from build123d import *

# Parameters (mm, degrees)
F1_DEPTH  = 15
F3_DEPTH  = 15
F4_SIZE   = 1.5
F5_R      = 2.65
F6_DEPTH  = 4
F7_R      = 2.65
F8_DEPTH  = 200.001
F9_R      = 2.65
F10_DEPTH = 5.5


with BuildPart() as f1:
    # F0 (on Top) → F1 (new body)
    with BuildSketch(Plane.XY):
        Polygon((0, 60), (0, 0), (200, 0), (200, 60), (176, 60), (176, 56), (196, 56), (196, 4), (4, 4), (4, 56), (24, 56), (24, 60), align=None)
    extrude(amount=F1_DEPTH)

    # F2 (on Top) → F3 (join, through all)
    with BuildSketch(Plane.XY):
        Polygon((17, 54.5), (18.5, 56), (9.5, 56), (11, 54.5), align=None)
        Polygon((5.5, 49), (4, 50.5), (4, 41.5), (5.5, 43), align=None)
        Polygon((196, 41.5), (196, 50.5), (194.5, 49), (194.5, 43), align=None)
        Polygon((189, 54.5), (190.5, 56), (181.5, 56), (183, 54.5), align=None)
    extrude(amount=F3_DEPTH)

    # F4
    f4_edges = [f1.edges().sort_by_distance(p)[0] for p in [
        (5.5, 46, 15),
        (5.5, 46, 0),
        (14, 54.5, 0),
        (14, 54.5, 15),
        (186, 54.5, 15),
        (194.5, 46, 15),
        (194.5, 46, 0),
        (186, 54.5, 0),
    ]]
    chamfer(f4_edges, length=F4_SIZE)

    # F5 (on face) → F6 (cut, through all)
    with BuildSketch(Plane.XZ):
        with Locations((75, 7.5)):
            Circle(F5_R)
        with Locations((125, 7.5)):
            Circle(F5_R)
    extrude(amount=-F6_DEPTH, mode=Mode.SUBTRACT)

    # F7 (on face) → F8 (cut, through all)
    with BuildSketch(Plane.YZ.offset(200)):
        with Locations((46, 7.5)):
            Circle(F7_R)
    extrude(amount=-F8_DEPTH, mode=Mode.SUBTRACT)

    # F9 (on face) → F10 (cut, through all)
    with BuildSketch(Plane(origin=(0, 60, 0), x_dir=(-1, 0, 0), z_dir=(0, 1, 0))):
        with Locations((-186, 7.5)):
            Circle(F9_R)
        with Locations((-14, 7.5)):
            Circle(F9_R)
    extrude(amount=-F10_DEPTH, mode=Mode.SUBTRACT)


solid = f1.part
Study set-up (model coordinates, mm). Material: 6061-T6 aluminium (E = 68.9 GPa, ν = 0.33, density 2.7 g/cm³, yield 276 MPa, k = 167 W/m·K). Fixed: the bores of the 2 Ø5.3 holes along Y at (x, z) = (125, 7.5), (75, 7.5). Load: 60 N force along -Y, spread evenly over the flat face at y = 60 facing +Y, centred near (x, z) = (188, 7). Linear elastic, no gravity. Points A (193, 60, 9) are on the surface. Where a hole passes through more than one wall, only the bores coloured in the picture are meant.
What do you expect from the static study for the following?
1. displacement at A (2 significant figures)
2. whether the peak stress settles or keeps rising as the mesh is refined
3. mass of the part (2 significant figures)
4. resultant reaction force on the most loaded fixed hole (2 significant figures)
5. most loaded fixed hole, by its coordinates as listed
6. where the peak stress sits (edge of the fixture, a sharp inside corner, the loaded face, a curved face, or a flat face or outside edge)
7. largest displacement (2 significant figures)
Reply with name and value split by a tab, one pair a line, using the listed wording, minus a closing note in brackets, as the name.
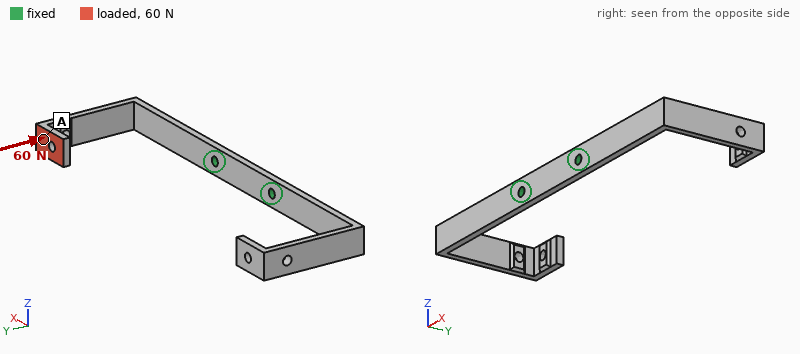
displacement at A	1.4 mm
whether the peak stress settles or keeps rising as the mesh is refined	keeps rising
mass of the part	57 g
resultant reaction force on the most loaded fixed hole	60 N
most loaded fixed hole, by its coordinates as listed	(125, 7.5)
where the peak stress sits	edge of the fixture
largest displacement	1.5 mm
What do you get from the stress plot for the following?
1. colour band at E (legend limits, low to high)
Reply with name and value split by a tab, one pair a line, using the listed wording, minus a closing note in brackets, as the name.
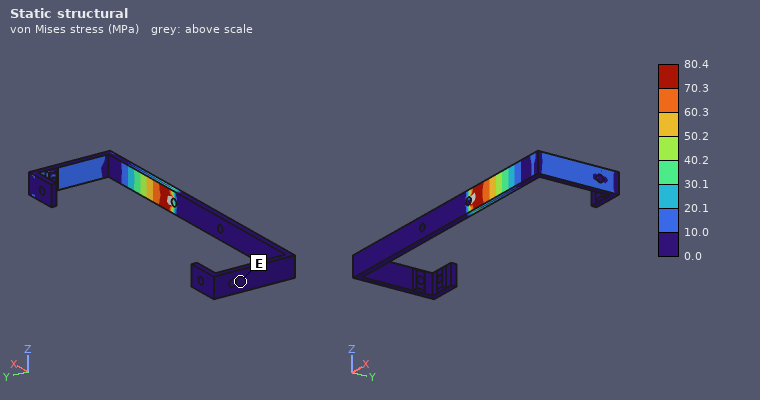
colour band at E	0.0 to 10.0 MPa
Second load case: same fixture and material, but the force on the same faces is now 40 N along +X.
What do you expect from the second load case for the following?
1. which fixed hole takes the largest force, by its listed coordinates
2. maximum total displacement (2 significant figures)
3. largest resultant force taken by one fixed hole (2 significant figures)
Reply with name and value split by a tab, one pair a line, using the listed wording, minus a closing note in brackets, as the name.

which fixed hole takes the largest force, by its listed coordinates	(125, 7.5)
maximum total displacement	2.4 mm
largest resultant force taken by one fixed hole	39 N
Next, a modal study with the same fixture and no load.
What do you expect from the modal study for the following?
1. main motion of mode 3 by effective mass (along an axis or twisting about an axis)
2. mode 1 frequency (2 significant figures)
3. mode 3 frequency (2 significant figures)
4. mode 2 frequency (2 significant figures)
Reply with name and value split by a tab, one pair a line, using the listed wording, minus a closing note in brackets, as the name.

main motion of mode 3 by effective mass	along Z
mode 1 frequency	210 Hz
mode 3 frequency	340 Hz
mode 2 frequency	210 Hz
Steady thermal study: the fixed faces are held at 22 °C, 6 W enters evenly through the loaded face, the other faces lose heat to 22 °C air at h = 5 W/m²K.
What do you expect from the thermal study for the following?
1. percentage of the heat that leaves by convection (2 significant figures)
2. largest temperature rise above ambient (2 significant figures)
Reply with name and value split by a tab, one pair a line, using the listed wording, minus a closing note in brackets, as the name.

percentage of the heat that leaves by convection	17 %
largest temperature rise above ambient	72 K
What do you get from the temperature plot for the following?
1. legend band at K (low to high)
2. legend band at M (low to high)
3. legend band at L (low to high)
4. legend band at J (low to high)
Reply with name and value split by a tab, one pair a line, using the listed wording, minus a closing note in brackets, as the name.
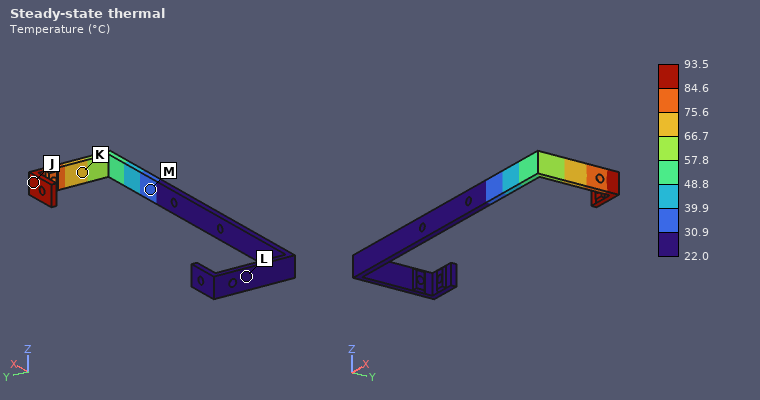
legend band at K	66.7 to 75.6 °C
legend band at M	30.9 to 39.9 °C
legend band at L	22.0 to 30.9 °C
legend band at J	84.6 to 93.5 °C
